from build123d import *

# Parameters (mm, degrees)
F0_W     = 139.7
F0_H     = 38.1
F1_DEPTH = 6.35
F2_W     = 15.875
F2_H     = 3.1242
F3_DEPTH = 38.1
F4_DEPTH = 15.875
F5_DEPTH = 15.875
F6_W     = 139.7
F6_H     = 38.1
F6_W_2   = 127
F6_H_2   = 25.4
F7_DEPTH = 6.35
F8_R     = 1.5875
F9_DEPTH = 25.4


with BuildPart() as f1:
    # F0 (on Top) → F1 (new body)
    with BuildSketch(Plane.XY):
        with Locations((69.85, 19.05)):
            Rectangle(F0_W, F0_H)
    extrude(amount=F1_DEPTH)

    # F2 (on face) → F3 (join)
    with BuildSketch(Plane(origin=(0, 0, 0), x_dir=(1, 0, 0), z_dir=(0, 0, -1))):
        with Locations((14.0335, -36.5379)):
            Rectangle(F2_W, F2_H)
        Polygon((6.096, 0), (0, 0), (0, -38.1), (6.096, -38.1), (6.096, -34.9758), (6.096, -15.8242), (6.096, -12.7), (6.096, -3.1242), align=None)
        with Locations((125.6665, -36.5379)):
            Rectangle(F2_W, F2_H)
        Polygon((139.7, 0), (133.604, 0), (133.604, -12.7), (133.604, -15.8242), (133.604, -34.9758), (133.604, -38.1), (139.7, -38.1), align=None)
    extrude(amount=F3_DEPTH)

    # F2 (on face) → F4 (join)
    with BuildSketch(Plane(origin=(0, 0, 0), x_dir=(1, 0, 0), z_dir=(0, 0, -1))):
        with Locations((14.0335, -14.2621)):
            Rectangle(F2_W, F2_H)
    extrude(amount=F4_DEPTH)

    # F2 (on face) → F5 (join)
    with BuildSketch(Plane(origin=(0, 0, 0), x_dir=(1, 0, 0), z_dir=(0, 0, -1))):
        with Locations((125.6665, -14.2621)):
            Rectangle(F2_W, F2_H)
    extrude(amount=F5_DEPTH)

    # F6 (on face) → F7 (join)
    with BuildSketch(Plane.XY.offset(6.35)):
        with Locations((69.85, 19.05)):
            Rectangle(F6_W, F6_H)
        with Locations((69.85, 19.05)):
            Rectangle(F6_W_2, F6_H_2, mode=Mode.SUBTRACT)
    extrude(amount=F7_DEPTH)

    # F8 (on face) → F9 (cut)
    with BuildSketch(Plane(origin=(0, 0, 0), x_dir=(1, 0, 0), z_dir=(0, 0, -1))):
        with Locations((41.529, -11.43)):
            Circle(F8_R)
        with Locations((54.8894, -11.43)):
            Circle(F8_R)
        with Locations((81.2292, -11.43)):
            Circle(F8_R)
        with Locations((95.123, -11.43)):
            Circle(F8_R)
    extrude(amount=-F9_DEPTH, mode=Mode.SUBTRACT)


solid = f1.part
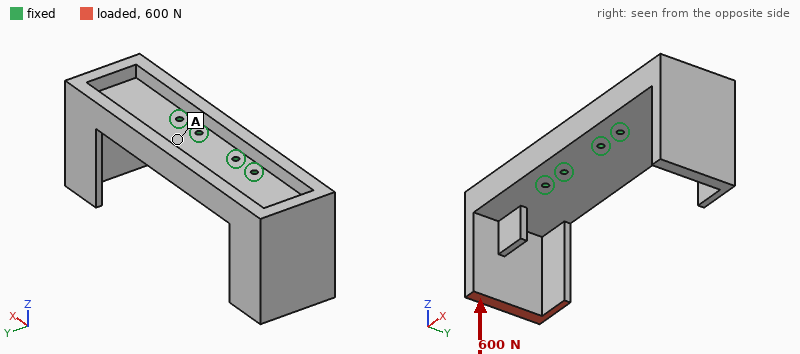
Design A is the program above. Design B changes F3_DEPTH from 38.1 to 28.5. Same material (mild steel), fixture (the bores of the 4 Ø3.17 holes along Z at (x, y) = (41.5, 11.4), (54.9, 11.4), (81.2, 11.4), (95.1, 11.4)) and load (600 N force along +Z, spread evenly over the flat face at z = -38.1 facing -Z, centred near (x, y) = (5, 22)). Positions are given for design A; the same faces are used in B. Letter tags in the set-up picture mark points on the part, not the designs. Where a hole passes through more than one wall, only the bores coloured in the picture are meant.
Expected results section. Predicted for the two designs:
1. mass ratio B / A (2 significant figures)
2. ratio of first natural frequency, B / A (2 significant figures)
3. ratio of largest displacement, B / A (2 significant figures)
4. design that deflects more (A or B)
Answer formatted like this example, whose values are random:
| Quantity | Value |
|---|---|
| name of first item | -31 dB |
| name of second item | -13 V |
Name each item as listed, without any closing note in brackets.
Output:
| Quantity | Value |
|---|---|
| mass ratio B / A | 0.92 |
| ratio of first natural frequency, B / A | 1.2 |
| ratio of largest displacement, B / A | 0.90 |
| design that deflects more | A |
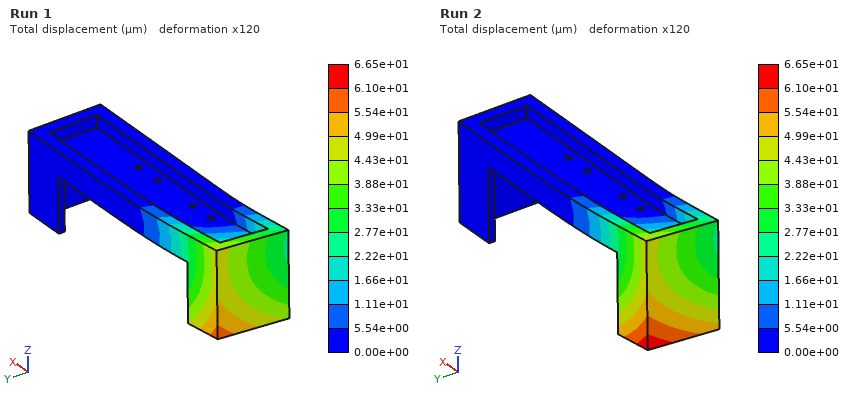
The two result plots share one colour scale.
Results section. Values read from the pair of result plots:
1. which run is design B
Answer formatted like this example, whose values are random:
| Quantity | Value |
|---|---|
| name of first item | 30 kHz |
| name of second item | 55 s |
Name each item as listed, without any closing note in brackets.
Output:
| Quantity | Value |
|---|---|
| which run is design B | Run 1 |
